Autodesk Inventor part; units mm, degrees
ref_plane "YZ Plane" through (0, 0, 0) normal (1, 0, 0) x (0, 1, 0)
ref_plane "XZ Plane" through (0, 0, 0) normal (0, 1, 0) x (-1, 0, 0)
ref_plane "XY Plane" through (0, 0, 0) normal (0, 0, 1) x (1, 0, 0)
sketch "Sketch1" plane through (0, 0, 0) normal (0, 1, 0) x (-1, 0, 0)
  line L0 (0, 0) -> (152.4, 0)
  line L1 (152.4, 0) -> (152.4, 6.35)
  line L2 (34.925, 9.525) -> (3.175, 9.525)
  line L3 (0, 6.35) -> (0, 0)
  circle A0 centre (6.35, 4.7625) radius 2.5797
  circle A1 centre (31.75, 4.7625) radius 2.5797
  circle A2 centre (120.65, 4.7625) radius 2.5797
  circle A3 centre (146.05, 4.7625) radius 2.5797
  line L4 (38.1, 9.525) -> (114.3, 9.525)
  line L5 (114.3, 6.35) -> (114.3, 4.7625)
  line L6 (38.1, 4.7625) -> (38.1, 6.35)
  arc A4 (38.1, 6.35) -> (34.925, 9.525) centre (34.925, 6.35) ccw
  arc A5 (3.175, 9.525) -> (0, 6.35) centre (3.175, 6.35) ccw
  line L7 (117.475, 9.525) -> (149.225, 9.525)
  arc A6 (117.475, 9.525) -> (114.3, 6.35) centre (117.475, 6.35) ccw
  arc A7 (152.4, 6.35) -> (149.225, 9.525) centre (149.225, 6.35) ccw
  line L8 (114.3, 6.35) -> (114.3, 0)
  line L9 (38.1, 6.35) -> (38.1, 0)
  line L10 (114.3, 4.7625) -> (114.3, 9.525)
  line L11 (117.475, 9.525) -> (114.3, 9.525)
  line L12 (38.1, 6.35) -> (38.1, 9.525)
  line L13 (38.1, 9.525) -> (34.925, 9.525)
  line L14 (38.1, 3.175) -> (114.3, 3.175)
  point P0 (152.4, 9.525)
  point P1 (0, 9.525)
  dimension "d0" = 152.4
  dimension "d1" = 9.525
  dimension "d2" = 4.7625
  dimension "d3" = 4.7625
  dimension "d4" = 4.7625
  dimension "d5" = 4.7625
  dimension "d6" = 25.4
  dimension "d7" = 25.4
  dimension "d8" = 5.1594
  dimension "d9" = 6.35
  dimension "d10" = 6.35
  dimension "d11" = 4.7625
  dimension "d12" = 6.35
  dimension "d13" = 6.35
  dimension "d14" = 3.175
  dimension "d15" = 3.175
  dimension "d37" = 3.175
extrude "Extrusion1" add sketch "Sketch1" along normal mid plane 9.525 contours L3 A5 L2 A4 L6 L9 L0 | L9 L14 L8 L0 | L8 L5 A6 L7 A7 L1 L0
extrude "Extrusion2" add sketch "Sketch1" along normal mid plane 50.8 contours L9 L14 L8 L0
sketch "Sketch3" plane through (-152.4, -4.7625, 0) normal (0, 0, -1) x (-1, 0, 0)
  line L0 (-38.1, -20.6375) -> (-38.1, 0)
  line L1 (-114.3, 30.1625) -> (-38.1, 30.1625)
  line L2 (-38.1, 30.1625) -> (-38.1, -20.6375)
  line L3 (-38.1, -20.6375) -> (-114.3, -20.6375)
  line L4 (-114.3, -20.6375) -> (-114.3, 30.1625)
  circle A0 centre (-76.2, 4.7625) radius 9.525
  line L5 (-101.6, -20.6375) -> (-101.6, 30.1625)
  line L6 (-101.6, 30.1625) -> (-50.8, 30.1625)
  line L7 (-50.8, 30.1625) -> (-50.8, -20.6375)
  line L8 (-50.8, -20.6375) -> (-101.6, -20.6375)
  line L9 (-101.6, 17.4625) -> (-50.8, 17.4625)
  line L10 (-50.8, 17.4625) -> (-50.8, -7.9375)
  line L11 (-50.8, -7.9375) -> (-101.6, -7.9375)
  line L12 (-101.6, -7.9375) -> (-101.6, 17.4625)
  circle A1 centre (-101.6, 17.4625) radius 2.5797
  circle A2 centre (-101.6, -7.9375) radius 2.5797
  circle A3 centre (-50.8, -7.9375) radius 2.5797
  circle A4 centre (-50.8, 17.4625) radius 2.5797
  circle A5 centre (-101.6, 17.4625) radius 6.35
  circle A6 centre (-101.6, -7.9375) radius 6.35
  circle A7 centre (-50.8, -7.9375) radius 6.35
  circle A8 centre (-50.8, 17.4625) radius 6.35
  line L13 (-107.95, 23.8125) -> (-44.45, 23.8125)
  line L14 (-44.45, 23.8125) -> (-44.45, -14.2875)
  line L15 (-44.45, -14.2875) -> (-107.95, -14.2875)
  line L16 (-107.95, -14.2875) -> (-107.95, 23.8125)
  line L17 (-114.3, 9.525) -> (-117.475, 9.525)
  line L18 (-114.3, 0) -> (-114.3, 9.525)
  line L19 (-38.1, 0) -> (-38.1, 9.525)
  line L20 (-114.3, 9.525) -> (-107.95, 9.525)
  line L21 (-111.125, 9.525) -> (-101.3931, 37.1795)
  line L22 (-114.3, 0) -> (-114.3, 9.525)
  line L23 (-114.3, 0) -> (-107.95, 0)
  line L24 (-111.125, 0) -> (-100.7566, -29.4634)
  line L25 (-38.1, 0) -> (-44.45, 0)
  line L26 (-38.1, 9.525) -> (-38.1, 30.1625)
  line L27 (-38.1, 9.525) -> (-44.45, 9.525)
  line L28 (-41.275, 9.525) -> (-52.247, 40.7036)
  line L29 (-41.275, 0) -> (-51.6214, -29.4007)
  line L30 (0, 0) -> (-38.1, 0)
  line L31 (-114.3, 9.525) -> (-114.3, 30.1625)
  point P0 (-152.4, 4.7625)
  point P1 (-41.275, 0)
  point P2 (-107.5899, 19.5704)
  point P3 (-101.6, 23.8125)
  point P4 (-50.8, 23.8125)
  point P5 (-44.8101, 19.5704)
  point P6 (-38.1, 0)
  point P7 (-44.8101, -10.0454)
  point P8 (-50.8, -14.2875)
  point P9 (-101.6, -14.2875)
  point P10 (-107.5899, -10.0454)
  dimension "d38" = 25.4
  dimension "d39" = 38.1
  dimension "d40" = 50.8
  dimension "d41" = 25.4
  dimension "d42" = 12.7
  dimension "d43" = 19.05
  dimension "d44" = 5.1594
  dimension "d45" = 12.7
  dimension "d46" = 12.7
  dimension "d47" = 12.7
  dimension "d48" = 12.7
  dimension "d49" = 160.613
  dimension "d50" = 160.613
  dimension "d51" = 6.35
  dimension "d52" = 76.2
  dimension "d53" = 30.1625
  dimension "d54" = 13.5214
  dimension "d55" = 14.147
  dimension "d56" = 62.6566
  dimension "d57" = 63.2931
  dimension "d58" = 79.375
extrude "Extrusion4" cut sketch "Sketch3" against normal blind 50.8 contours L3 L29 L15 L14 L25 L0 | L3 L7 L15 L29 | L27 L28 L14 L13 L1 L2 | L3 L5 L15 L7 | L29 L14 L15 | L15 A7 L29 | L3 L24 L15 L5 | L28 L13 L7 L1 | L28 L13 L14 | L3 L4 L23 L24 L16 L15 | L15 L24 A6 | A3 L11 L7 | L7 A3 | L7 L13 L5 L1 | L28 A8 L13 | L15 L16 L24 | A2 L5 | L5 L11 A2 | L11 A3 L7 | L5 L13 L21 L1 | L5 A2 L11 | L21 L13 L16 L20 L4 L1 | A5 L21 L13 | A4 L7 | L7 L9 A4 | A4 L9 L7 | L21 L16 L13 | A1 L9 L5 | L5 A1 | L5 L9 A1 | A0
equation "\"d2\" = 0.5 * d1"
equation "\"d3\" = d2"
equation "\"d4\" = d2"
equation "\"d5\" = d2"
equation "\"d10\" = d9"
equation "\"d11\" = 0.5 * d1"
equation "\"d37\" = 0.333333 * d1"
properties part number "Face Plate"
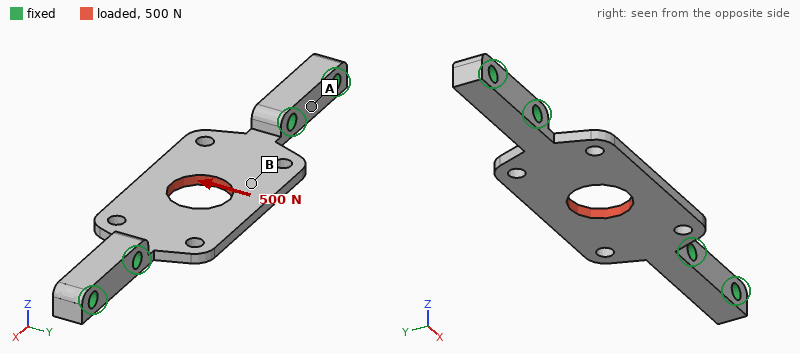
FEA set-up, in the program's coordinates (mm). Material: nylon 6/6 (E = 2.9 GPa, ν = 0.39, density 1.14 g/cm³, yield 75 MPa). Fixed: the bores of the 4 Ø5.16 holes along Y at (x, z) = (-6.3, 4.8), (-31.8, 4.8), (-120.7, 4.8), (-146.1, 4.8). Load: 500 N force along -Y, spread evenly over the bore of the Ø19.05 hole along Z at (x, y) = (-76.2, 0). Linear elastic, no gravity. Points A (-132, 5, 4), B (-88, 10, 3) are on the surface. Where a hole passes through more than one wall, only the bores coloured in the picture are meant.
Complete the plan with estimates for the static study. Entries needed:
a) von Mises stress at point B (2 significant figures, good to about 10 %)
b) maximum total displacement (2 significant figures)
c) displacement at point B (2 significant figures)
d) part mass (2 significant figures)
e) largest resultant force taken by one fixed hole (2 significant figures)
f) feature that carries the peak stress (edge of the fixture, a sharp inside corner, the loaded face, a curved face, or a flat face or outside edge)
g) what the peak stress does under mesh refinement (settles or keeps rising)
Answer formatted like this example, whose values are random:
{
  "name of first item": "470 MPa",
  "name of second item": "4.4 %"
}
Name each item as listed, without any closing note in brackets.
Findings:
{
  "von Mises stress at point B": "6.2 MPa",
  "maximum total displacement": "0.28 mm",
  "displacement at point B": "0.25 mm",
  "part mass": "15 g",
  "largest resultant force taken by one fixed hole": "250 N",
  "feature that carries the peak stress": "edge of the fixture",
  "what the peak stress does under mesh refinement": "keeps rising"
}
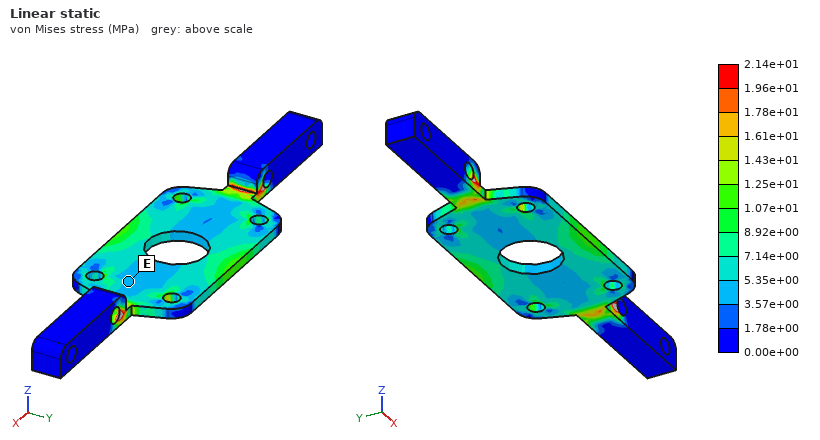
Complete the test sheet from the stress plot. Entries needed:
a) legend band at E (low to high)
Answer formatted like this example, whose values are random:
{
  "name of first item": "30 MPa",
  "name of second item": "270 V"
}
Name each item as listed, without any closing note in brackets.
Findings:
{
  "legend band at E": "3.57e+00 to 5.35e+00 MPa"
}
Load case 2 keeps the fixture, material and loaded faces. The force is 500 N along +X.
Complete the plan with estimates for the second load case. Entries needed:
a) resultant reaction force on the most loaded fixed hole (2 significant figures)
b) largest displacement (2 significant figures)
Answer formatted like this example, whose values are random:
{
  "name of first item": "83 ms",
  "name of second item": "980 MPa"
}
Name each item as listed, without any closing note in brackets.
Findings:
{
  "resultant reaction force on the most loaded fixed hole": "250 N",
  "largest displacement": "72 µm"
}
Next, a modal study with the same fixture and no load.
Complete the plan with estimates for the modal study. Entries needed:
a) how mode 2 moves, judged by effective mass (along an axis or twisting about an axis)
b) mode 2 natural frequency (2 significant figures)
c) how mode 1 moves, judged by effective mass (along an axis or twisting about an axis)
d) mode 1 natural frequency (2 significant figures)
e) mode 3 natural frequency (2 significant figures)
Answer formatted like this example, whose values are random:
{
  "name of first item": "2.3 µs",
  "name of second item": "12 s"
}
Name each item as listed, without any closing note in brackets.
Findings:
{
  "how mode 2 moves, judged by effective mass": "twisting about X",
  "mode 2 natural frequency": "690 Hz",
  "how mode 1 moves, judged by effective mass": "along Z",
  "mode 1 natural frequency": "580 Hz",
  "mode 3 natural frequency": "1600 Hz"
}
